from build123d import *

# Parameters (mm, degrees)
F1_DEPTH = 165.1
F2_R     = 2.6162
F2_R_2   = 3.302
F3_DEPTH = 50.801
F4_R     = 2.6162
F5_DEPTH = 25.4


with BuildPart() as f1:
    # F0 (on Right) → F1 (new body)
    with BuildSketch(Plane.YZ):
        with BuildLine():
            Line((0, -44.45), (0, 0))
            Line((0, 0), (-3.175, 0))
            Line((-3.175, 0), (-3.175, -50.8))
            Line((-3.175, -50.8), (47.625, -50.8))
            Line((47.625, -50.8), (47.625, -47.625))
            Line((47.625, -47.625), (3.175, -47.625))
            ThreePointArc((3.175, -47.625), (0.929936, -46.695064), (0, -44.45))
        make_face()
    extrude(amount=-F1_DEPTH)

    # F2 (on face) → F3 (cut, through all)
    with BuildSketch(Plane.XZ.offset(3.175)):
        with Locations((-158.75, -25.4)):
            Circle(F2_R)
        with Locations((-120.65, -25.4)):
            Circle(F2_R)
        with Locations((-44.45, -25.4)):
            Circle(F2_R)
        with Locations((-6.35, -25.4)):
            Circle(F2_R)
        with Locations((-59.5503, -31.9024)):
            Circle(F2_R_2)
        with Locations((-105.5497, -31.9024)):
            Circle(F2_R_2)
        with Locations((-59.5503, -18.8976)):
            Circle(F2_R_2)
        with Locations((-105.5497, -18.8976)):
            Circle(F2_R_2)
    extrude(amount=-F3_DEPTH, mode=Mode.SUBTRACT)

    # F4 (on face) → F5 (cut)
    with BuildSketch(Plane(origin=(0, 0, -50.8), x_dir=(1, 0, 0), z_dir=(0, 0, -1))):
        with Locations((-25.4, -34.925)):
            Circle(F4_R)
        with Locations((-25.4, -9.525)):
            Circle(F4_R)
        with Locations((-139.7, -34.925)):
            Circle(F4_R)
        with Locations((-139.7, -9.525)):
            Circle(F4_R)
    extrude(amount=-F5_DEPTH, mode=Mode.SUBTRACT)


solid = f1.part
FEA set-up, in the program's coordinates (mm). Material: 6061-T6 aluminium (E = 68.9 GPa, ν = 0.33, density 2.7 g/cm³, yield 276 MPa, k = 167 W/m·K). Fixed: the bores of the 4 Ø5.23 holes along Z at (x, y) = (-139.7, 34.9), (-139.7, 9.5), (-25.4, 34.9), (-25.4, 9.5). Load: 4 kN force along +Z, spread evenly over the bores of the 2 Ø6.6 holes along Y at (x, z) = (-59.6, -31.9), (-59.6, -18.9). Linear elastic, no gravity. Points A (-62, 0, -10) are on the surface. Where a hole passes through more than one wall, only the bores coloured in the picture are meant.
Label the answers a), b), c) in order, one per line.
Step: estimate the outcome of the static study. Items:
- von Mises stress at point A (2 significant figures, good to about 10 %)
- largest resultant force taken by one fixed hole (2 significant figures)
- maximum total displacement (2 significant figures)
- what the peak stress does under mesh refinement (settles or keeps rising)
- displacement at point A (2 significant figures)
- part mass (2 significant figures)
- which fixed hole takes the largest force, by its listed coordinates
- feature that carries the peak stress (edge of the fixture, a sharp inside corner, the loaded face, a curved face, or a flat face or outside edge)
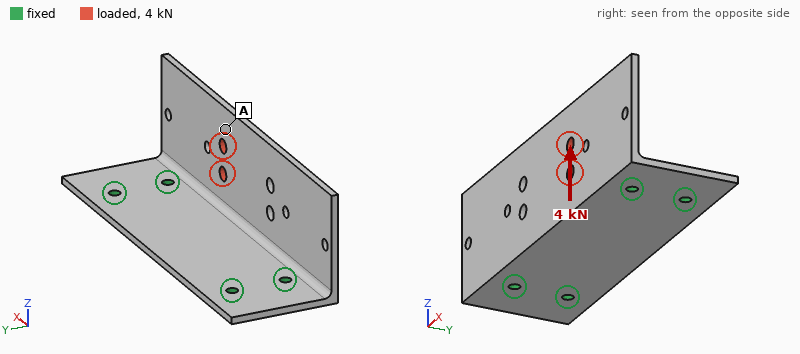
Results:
a) 38 MPa
b) 3.5 kN
c) 0.84 mm
d) keeps rising
e) 0.52 mm
f) 140 g
g) (-25.4, 9.5)
h) edge of the fixture
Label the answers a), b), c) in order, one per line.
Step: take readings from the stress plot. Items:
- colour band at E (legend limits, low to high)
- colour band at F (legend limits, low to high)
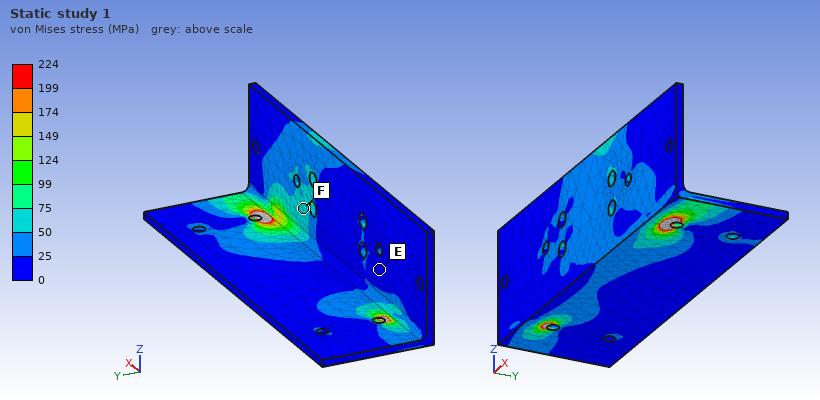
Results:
a) 0 to 25 MPa
b) 50 to 75 MPa
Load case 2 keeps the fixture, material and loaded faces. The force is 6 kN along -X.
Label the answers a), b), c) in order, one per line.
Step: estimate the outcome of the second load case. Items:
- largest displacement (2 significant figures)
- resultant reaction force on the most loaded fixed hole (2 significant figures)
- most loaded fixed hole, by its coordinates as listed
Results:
a) 0.34 mm
b) 3.0 kN
c) (-25.4, 9.5)
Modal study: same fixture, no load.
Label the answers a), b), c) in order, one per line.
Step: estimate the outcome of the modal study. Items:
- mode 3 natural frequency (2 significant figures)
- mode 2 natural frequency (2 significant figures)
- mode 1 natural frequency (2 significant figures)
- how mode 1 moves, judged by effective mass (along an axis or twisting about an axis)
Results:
a) 1600 Hz
b) 1100 Hz
c) 770 Hz
d) along Y
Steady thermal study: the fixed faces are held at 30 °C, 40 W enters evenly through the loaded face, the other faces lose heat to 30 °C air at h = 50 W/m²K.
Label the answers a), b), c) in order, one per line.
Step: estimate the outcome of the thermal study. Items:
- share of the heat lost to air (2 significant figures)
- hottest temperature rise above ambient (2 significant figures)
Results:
a) 41 %
b) 40 K
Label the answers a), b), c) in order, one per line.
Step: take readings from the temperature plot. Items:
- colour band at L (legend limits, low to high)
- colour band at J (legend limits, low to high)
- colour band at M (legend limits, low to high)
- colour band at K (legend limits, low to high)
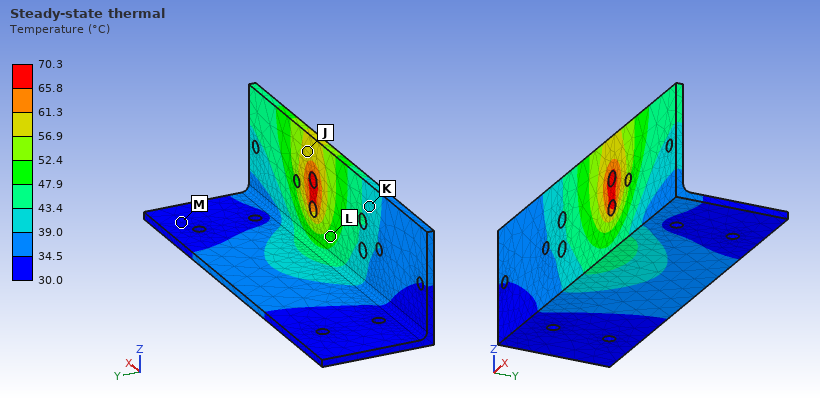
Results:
a) 47.9 to 52.4 °C
b) 56.9 to 61.3 °C
c) 30.0 to 34.5 °C
d) 39.0 to 43.4 °C
